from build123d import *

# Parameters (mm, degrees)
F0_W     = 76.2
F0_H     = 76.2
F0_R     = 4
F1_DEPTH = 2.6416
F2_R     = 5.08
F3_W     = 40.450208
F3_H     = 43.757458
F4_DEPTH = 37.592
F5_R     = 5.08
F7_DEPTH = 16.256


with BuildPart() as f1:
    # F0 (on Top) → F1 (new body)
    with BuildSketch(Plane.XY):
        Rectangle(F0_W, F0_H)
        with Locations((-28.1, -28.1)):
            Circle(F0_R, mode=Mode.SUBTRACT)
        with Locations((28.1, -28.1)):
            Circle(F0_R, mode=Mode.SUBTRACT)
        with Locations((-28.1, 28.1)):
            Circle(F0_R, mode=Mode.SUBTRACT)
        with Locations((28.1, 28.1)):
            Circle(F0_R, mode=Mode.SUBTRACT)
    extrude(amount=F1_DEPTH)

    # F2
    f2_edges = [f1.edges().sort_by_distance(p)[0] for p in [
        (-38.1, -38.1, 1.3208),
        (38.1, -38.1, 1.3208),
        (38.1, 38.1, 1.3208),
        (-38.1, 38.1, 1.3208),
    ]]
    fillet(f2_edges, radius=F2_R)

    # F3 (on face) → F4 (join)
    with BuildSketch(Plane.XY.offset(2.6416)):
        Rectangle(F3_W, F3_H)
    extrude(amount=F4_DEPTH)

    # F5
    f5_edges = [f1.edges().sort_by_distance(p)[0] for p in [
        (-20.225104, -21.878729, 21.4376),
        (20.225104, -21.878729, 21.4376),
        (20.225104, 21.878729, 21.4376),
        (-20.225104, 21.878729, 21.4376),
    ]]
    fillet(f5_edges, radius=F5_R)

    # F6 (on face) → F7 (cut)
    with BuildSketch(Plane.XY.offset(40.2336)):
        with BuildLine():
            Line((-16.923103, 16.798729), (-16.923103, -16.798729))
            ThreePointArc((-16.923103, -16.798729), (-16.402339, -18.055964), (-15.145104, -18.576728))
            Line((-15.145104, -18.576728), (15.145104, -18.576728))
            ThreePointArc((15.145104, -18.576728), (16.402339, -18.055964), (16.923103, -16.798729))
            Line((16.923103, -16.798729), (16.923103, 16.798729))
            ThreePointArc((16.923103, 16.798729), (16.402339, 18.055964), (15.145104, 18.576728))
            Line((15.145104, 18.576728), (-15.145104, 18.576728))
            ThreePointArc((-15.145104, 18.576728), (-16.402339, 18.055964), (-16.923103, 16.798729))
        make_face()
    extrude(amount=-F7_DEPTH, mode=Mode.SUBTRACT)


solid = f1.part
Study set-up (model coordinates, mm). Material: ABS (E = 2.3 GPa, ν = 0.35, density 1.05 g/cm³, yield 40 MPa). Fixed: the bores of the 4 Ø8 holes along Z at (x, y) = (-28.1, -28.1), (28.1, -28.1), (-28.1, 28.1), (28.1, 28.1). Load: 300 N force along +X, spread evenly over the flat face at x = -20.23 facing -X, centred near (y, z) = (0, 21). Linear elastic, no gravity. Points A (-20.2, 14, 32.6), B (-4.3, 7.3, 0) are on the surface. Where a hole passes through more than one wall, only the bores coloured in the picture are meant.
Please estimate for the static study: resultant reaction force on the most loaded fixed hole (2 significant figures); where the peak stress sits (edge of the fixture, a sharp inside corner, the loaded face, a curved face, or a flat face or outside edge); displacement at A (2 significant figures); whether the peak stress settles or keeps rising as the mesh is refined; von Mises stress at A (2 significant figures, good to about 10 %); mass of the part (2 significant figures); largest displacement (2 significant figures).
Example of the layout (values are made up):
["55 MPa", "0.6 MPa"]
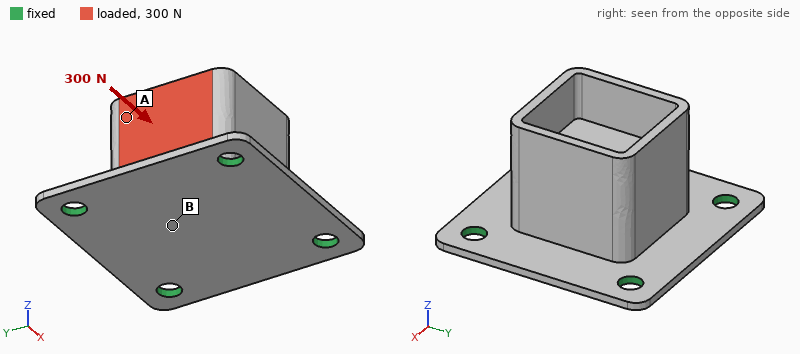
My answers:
["110 N", "edge of the fixture", "0.29 mm", "keeps rising", "4.2 MPa", "63 g", "0.48 mm"]
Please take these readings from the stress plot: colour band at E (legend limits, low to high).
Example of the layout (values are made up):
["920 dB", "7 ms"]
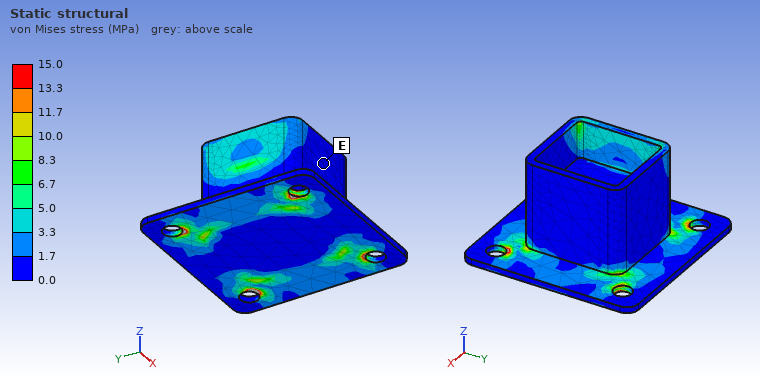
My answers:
["0.0 to 1.7 MPa"]
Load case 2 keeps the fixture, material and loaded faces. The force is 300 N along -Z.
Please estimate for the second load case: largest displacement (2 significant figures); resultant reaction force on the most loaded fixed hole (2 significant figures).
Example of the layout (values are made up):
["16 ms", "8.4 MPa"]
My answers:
["0.43 mm", "150 N"]
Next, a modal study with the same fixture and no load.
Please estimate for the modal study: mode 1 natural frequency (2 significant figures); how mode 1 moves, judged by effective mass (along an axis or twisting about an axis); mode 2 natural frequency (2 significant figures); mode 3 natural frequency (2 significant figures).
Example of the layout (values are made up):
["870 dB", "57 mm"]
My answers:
["920 Hz", "along Z", "980 Hz", "980 Hz"]
